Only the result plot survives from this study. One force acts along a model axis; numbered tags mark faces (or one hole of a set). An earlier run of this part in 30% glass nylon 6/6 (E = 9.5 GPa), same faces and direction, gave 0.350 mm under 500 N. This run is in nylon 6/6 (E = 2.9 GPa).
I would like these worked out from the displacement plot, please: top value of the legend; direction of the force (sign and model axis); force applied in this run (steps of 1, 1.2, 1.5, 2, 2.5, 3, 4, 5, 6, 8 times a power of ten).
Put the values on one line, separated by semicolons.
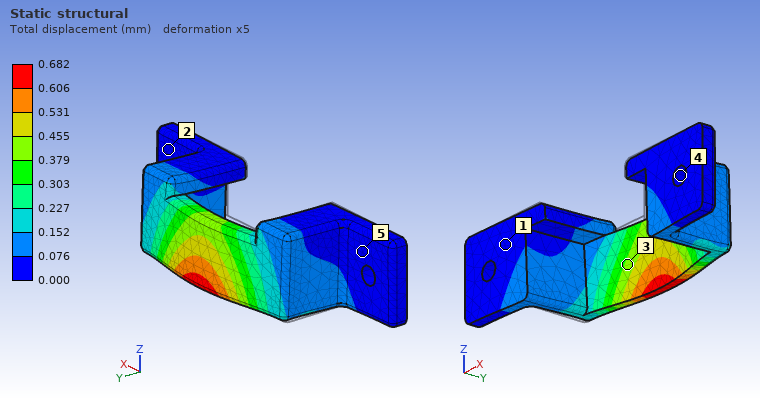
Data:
0.682 mm; +Y; 300 N
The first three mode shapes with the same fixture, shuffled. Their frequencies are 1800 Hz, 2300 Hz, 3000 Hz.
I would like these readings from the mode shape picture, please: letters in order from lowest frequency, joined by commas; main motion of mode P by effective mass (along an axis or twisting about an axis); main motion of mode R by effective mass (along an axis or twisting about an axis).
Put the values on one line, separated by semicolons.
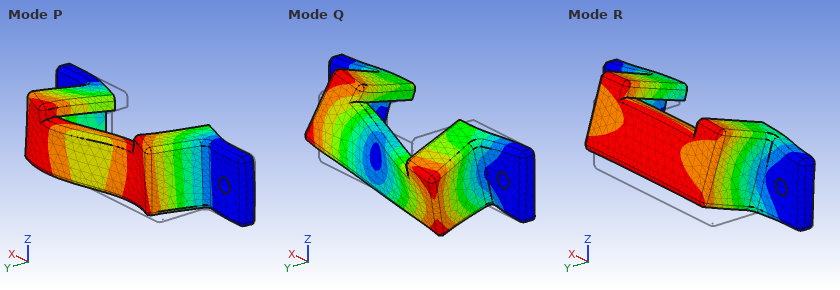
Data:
R, P, Q; along X; along Z
